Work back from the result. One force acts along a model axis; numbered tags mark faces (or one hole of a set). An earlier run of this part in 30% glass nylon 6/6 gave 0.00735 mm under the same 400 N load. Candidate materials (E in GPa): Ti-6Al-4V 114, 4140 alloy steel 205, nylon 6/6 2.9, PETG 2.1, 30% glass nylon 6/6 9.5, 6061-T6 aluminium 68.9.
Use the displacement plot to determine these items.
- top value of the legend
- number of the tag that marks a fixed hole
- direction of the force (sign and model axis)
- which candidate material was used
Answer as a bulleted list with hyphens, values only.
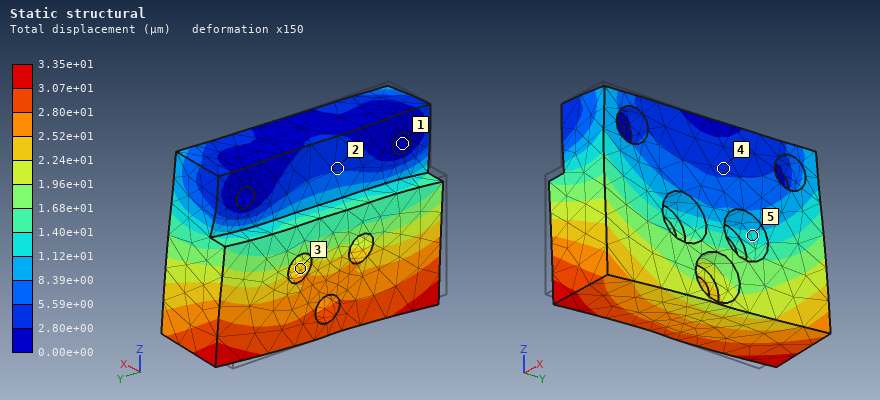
- 3.35e+01 µm
- 1
- +Y
- PETG
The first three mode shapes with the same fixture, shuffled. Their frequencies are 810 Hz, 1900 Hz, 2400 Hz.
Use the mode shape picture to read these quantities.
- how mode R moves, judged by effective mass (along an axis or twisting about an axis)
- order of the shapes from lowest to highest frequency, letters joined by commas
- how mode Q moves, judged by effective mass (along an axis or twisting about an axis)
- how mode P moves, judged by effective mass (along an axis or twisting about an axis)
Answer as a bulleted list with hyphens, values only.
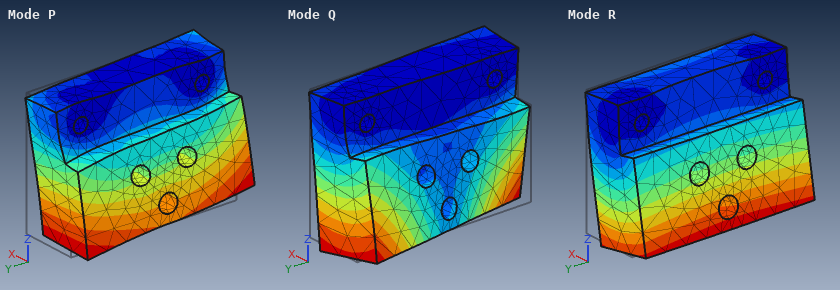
- along X
- R, Q, P
- twisting about Z
- along Y
